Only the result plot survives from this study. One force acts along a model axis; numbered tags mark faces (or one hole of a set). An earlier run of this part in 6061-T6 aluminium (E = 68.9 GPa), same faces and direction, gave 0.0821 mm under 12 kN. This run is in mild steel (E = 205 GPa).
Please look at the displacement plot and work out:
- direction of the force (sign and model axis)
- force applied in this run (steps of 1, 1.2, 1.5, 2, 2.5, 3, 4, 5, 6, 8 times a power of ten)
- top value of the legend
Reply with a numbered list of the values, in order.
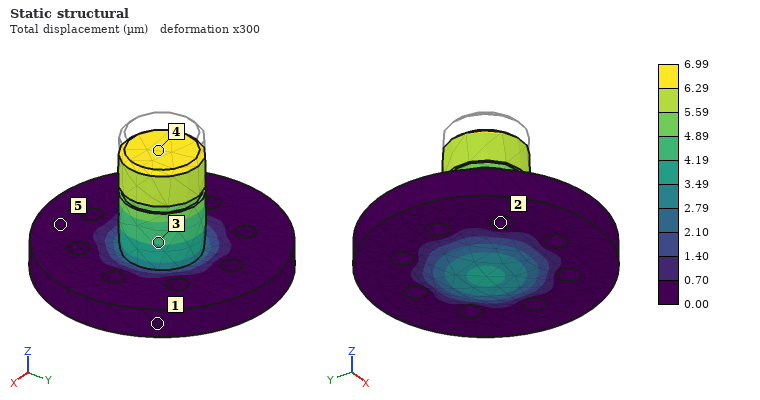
1. -Z
2. 3 kN
3. 6.99 µm
